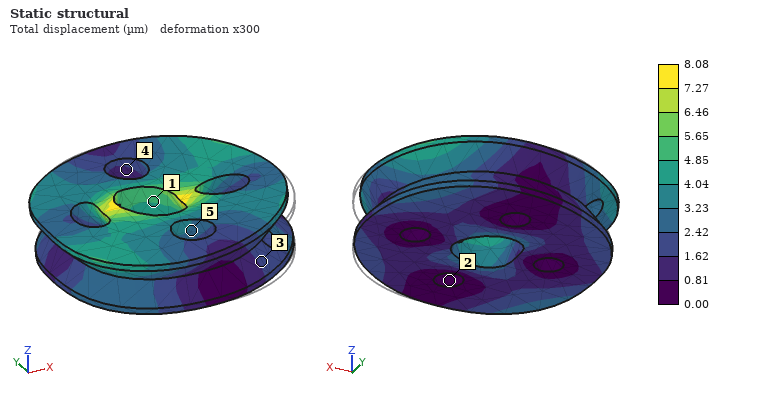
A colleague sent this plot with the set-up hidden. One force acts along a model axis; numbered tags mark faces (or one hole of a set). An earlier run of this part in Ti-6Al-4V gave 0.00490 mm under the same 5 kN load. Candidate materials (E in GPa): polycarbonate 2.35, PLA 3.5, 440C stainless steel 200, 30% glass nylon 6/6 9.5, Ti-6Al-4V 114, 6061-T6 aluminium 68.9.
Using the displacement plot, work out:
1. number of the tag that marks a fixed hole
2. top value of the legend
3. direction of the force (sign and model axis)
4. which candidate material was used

2
8.08 µm
-X
6061-T6 aluminium
